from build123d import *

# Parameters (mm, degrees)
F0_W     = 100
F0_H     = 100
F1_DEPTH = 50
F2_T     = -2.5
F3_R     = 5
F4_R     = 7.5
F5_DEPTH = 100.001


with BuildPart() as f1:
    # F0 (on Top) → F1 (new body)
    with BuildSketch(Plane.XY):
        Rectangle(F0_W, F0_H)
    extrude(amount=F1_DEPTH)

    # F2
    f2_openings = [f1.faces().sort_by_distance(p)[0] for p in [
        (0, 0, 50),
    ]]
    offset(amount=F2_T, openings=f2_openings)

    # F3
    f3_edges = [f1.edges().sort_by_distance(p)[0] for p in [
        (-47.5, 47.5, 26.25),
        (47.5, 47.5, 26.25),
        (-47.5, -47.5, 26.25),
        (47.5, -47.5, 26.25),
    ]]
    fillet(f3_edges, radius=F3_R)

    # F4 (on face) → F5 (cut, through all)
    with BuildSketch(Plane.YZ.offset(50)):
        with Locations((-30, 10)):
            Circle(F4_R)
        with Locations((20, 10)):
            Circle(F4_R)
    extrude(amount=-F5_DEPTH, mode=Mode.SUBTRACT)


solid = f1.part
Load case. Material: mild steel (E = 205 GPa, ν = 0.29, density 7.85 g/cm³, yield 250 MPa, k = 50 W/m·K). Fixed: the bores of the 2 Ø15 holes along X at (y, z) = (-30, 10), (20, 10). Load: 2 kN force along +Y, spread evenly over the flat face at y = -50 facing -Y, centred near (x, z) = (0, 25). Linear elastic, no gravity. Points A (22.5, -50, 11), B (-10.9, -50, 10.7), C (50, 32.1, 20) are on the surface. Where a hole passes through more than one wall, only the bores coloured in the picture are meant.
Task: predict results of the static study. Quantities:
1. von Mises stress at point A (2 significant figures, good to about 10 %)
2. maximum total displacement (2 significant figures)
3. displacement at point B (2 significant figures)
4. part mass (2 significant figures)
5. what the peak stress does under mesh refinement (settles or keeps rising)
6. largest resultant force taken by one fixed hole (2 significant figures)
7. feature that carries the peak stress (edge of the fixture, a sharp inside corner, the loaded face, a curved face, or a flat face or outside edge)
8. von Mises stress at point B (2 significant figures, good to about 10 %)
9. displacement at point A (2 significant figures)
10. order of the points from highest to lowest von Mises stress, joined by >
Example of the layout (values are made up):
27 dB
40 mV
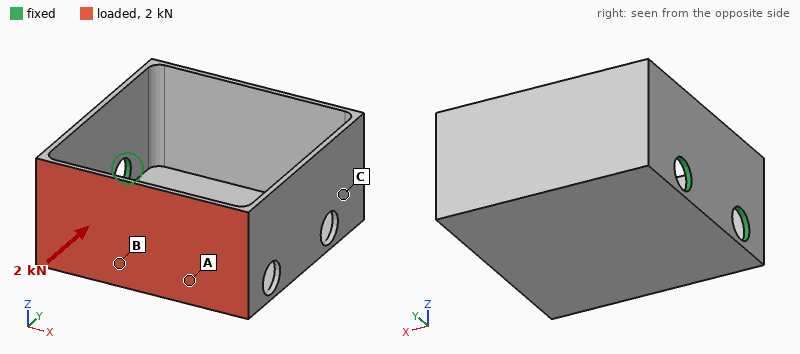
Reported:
43 MPa
0.64 mm
0.11 mm
550 g
keeps rising
2.3 kN
edge of the fixture
80 MPa
0.16 mm
B > A > C
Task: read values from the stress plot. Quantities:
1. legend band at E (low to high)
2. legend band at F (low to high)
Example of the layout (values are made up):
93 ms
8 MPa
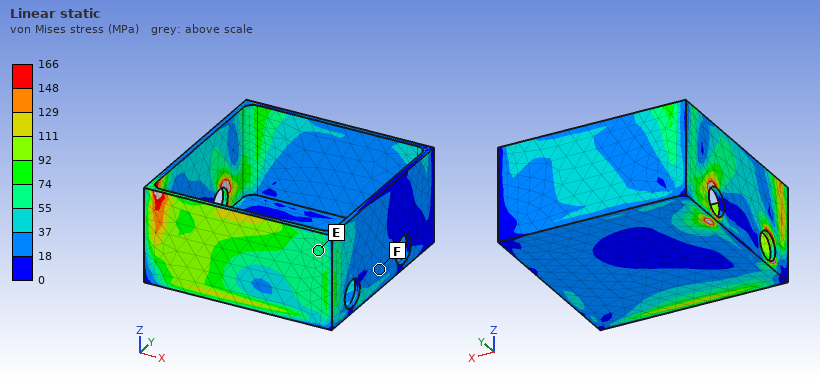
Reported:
55 to 74 MPa
18 to 37 MPa
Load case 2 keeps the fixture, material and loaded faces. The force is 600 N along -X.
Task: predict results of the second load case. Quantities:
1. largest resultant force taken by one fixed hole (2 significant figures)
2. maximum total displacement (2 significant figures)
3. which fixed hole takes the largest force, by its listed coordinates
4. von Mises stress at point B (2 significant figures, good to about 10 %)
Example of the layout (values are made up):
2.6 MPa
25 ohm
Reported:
720 N
0.19 mm
(-30, 10)
11 MPa
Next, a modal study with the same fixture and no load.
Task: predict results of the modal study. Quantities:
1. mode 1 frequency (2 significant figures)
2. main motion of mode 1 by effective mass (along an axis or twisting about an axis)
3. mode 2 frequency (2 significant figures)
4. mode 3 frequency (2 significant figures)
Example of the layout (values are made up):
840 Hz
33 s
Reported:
300 Hz
along Z
490 Hz
1400 Hz
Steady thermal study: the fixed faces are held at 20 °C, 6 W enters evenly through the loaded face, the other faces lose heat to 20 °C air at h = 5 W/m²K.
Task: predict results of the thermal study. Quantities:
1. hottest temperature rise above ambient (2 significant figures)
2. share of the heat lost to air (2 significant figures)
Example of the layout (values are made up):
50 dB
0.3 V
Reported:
19 K
29 %
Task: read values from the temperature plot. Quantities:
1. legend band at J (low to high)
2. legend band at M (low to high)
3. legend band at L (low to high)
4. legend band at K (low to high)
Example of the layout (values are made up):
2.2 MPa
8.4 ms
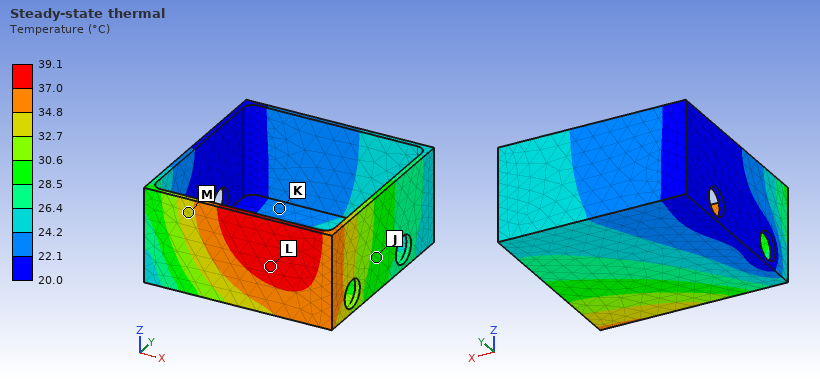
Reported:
28.5 to 30.6 °C
32.7 to 34.8 °C
37.0 to 39.1 °C
22.1 to 24.2 °C
